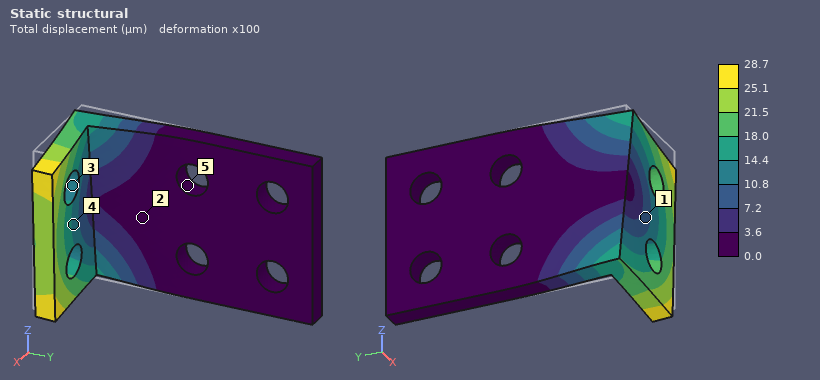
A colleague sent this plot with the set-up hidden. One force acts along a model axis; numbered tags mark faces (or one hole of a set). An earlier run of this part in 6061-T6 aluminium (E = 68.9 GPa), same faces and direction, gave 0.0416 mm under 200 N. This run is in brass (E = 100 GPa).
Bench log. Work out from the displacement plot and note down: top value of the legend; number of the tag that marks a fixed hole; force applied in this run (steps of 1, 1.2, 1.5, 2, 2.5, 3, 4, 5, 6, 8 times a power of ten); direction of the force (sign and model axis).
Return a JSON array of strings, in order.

["28.7 µm", "5", "200 N", "-Z"]
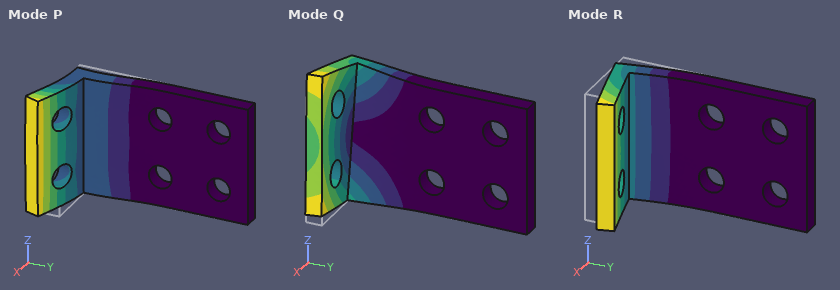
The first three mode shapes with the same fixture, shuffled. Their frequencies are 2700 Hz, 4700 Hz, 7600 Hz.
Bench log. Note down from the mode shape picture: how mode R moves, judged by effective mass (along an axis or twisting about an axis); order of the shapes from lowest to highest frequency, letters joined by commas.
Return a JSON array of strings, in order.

["along X", "R, Q, P"]
